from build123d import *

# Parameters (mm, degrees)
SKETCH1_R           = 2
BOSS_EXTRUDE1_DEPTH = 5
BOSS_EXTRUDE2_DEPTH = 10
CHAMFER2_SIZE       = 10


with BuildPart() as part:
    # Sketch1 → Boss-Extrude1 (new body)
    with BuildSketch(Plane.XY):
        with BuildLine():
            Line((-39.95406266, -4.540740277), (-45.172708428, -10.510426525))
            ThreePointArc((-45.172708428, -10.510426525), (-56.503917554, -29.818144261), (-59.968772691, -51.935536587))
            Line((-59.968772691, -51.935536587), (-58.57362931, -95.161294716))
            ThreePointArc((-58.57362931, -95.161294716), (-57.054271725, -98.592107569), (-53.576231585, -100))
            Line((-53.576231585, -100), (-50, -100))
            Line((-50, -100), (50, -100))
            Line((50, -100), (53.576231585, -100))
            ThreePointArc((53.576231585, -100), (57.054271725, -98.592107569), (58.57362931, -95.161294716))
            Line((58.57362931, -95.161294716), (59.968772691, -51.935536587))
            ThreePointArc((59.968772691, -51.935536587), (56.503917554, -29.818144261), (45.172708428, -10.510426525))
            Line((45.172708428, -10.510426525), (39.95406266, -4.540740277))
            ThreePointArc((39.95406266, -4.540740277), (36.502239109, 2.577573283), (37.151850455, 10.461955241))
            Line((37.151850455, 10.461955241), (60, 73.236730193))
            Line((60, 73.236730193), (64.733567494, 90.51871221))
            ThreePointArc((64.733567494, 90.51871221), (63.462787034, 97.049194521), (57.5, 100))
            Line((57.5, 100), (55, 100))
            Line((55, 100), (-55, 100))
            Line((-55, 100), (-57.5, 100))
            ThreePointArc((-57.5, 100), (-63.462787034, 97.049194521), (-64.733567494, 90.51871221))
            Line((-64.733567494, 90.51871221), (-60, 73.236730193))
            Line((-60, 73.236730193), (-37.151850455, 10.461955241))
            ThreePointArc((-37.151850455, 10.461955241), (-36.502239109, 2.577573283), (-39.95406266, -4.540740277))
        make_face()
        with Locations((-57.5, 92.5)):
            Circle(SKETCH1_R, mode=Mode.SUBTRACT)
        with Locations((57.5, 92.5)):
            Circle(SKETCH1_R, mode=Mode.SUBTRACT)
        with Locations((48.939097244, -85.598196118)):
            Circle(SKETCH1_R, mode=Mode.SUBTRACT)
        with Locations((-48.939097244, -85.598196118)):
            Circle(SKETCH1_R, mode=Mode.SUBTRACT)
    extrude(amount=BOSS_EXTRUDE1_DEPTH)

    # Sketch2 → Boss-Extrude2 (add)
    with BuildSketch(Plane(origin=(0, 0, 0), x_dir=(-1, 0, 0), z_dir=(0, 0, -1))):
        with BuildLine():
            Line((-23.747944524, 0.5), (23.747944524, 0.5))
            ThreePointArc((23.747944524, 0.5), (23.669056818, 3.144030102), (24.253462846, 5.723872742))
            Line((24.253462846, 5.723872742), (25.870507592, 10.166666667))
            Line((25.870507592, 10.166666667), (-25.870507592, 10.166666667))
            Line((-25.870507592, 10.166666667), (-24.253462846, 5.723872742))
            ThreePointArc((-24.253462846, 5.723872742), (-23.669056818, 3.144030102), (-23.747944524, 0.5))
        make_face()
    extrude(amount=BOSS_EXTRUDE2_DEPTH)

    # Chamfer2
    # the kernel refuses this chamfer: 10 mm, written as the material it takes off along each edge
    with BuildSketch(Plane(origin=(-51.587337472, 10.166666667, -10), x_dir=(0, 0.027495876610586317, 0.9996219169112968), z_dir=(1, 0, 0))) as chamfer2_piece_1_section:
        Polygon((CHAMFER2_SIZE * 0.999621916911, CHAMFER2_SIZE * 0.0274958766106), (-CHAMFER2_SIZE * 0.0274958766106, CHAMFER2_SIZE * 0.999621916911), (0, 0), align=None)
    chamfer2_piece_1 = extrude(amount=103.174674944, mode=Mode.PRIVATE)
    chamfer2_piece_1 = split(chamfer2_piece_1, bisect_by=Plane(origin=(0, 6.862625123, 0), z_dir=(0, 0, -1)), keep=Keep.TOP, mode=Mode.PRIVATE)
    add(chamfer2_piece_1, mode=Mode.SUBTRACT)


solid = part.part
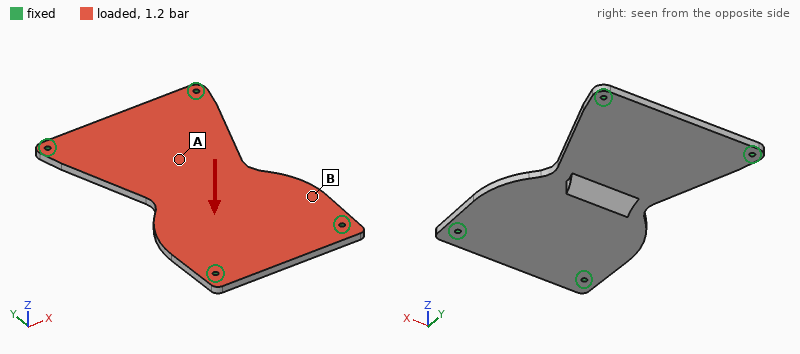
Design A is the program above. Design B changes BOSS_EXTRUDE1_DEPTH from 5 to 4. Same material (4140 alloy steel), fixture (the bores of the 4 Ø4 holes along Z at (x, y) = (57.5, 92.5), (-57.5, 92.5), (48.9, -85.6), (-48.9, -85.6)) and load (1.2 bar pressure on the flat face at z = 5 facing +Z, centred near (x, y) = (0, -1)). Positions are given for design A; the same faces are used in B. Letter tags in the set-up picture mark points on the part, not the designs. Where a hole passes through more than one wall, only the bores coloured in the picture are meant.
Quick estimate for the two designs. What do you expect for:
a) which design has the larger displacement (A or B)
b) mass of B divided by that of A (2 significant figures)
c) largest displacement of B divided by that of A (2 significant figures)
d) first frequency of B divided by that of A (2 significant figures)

B
0.80
1.9
0.81
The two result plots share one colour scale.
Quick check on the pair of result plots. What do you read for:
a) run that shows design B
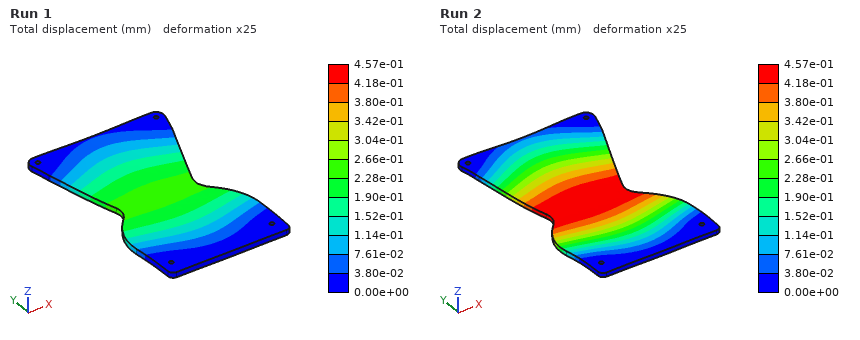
Run 2
